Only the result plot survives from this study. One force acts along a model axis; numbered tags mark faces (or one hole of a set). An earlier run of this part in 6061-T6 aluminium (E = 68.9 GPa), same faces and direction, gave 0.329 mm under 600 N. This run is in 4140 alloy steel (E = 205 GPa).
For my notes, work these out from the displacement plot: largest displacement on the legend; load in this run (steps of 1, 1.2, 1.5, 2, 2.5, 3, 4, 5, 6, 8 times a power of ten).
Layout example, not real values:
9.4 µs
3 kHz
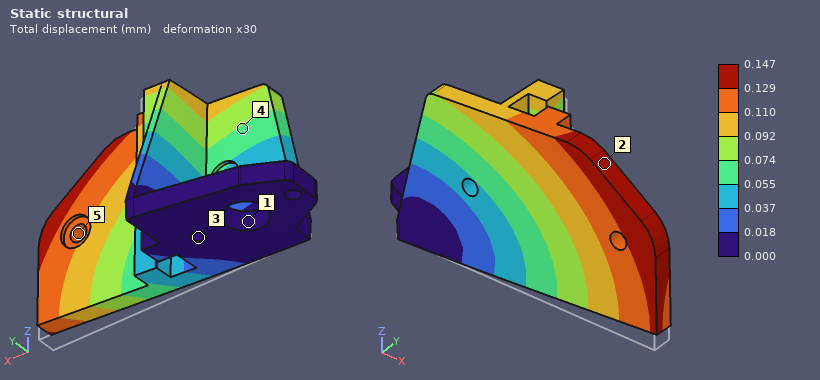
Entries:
0.147 mm
800 N
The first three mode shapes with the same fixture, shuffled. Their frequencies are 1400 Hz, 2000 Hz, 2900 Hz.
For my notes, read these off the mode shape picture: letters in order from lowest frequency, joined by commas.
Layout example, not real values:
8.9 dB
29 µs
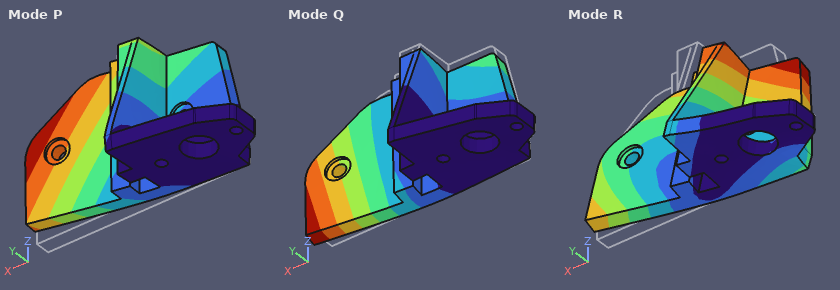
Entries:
P, Q, R
